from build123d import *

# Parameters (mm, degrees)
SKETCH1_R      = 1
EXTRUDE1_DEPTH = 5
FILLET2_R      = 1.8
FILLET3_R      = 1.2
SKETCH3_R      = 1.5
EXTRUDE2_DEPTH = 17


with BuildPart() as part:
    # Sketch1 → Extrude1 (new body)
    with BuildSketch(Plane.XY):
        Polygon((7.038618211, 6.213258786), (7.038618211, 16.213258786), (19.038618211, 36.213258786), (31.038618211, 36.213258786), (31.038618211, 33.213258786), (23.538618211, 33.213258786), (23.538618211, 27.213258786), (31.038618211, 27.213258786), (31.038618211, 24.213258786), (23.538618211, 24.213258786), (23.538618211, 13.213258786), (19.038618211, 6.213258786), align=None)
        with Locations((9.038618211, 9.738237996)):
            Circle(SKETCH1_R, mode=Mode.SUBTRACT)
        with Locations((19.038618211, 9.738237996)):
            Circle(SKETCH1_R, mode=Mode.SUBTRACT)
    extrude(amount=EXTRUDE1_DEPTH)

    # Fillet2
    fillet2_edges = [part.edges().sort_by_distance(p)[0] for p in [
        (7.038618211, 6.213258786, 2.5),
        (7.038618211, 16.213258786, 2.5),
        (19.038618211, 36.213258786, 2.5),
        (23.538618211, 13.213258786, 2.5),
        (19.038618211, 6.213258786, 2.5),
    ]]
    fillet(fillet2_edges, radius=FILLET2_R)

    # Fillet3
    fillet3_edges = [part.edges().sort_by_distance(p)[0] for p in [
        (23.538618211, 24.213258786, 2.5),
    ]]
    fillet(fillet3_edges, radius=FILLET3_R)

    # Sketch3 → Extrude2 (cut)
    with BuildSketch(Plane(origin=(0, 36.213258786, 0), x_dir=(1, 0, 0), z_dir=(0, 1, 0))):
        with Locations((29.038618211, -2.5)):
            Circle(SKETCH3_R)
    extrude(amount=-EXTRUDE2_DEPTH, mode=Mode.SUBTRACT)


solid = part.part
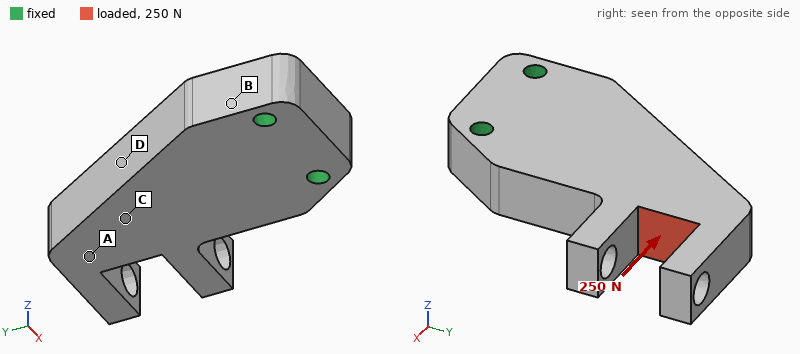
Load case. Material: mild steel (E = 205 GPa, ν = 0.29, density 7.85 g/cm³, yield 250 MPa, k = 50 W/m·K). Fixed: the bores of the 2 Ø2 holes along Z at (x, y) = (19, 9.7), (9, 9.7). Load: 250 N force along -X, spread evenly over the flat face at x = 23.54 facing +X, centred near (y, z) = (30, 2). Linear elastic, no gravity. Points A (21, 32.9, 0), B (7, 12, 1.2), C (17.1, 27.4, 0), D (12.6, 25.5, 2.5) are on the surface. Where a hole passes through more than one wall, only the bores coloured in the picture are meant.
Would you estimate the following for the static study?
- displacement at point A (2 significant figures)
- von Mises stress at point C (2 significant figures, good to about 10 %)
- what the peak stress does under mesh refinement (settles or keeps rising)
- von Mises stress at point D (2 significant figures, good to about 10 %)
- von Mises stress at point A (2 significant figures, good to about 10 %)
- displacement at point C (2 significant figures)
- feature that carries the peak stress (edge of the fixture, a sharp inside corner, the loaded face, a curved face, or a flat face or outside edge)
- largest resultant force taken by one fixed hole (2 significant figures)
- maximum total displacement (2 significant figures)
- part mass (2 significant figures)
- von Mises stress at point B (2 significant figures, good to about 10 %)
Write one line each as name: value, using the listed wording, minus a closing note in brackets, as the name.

displacement at point A: 5.0 µm
von Mises stress at point C: 10 MPa
what the peak stress does under mesh refinement: keeps rising
von Mises stress at point D: 17 MPa
von Mises stress at point A: 4.6 MPa
displacement at point C: 3.1 µm
feature that carries the peak stress: edge of the fixture
largest resultant force taken by one fixed hole: 500 N
maximum total displacement: 6.7 µm
part mass: 15 g
von Mises stress at point B: 20 MPa
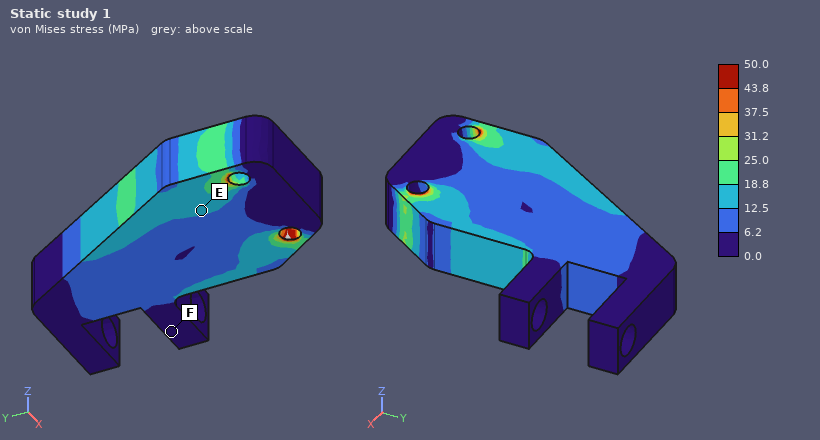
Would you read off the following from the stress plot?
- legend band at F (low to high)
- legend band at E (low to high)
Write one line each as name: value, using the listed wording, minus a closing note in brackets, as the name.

legend band at F: 0.0 to 6.2 MPa
legend band at E: 12.5 to 18.8 MPa
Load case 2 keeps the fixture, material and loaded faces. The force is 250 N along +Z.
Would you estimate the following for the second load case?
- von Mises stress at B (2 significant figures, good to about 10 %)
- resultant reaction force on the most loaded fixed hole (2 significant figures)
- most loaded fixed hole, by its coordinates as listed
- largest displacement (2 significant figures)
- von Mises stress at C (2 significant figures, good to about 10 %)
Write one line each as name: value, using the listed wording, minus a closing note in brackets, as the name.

von Mises stress at B: 32 MPa
resultant reaction force on the most loaded fixed hole: 300 N
most loaded fixed hole, by its coordinates as listed: (19, 9.7)
largest displacement: 52 µm
von Mises stress at C: 33 MPa
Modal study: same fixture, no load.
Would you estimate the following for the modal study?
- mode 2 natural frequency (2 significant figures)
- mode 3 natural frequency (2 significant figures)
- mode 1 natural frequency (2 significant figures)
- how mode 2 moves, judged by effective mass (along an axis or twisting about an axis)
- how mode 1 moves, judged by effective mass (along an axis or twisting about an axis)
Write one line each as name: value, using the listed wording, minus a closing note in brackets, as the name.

mode 2 natural frequency: 15 kHz
mode 3 natural frequency: 20 kHz
mode 1 natural frequency: 6100 Hz
how mode 2 moves, judged by effective mass: along X
how mode 1 moves, judged by effective mass: along Z
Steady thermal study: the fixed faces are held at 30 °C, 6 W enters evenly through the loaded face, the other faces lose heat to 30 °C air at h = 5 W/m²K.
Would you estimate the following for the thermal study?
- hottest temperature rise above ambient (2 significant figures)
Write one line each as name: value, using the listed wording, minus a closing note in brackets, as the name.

hottest temperature rise above ambient: 49 K
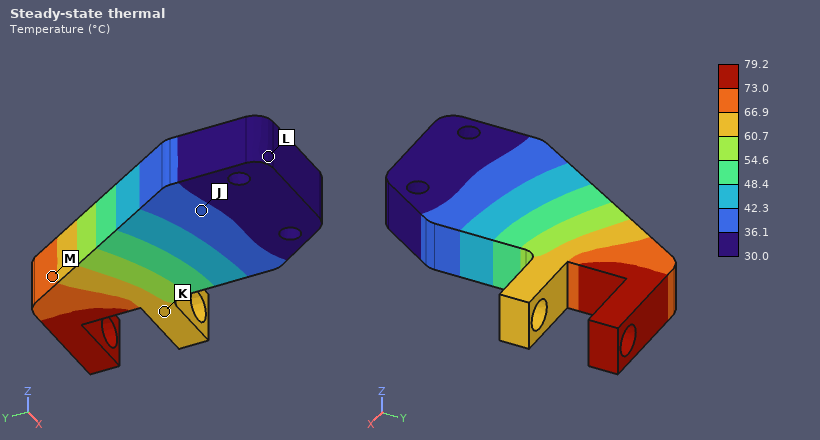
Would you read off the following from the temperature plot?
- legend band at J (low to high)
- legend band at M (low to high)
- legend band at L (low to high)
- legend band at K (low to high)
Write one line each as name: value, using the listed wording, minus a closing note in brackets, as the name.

legend band at J: 36.1 to 42.3 °C
legend band at M: 66.9 to 73.0 °C
legend band at L: 30.0 to 36.1 °C
legend band at K: 60.7 to 66.9 °C
